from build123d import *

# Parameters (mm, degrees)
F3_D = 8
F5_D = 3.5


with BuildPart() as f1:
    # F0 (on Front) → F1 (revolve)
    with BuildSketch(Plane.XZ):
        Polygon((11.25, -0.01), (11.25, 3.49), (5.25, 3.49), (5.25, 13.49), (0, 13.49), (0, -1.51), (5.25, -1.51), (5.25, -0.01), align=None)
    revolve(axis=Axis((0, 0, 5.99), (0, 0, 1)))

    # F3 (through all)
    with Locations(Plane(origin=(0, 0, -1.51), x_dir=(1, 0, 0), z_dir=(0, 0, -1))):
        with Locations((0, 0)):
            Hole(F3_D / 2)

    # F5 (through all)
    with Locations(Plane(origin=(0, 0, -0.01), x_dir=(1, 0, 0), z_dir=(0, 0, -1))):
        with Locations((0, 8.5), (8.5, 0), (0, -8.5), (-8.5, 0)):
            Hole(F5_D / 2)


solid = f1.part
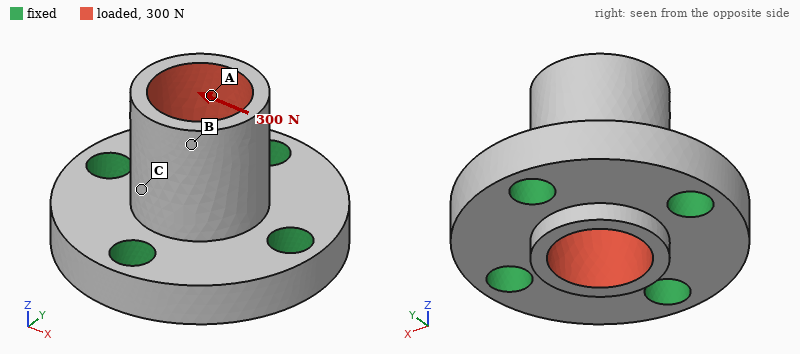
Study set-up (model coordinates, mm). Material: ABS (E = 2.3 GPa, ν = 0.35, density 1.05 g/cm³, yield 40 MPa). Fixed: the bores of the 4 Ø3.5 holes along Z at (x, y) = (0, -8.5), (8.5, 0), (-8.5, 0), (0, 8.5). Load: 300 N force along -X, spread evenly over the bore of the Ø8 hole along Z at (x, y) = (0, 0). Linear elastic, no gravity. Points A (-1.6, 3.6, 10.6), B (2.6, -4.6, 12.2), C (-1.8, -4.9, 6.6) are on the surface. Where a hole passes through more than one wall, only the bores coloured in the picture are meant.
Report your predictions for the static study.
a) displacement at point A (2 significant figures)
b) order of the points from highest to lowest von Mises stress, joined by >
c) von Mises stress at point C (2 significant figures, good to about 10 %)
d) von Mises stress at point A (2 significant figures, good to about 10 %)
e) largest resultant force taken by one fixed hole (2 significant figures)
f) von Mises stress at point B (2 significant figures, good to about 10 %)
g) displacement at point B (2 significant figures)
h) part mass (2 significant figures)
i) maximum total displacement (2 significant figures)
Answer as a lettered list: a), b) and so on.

a) 0.11 mm
b) C > A > B
c) 9.7 MPa
d) 6.0 MPa
e) 120 N
f) 2.4 MPa
g) 0.12 mm
h) 1.6 g
i) 0.14 mm
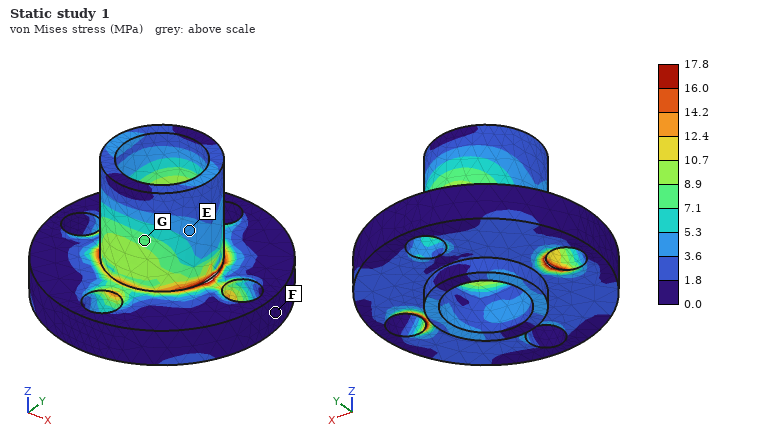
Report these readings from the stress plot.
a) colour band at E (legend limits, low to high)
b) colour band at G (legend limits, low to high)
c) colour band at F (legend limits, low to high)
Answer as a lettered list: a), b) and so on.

a) 3.6 to 5.3 MPa
b) 7.1 to 8.9 MPa
c) 0.0 to 1.8 MPa
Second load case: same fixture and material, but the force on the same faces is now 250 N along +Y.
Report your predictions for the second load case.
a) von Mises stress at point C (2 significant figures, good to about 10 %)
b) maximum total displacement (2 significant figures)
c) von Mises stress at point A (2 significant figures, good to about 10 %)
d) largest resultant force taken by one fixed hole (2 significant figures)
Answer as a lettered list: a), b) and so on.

a) 4.4 MPa
b) 0.12 mm
c) 3.9 MPa
d) 100 N
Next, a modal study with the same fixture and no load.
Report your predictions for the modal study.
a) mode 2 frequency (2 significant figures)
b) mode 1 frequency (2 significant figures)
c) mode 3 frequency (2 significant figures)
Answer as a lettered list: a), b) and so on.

a) 11 kHz
b) 11 kHz
c) 13 kHz
